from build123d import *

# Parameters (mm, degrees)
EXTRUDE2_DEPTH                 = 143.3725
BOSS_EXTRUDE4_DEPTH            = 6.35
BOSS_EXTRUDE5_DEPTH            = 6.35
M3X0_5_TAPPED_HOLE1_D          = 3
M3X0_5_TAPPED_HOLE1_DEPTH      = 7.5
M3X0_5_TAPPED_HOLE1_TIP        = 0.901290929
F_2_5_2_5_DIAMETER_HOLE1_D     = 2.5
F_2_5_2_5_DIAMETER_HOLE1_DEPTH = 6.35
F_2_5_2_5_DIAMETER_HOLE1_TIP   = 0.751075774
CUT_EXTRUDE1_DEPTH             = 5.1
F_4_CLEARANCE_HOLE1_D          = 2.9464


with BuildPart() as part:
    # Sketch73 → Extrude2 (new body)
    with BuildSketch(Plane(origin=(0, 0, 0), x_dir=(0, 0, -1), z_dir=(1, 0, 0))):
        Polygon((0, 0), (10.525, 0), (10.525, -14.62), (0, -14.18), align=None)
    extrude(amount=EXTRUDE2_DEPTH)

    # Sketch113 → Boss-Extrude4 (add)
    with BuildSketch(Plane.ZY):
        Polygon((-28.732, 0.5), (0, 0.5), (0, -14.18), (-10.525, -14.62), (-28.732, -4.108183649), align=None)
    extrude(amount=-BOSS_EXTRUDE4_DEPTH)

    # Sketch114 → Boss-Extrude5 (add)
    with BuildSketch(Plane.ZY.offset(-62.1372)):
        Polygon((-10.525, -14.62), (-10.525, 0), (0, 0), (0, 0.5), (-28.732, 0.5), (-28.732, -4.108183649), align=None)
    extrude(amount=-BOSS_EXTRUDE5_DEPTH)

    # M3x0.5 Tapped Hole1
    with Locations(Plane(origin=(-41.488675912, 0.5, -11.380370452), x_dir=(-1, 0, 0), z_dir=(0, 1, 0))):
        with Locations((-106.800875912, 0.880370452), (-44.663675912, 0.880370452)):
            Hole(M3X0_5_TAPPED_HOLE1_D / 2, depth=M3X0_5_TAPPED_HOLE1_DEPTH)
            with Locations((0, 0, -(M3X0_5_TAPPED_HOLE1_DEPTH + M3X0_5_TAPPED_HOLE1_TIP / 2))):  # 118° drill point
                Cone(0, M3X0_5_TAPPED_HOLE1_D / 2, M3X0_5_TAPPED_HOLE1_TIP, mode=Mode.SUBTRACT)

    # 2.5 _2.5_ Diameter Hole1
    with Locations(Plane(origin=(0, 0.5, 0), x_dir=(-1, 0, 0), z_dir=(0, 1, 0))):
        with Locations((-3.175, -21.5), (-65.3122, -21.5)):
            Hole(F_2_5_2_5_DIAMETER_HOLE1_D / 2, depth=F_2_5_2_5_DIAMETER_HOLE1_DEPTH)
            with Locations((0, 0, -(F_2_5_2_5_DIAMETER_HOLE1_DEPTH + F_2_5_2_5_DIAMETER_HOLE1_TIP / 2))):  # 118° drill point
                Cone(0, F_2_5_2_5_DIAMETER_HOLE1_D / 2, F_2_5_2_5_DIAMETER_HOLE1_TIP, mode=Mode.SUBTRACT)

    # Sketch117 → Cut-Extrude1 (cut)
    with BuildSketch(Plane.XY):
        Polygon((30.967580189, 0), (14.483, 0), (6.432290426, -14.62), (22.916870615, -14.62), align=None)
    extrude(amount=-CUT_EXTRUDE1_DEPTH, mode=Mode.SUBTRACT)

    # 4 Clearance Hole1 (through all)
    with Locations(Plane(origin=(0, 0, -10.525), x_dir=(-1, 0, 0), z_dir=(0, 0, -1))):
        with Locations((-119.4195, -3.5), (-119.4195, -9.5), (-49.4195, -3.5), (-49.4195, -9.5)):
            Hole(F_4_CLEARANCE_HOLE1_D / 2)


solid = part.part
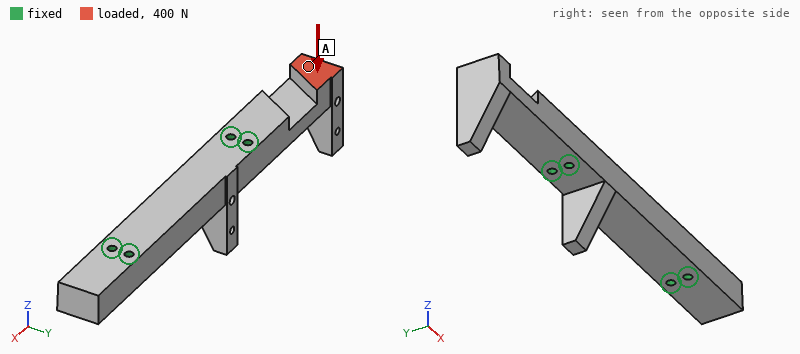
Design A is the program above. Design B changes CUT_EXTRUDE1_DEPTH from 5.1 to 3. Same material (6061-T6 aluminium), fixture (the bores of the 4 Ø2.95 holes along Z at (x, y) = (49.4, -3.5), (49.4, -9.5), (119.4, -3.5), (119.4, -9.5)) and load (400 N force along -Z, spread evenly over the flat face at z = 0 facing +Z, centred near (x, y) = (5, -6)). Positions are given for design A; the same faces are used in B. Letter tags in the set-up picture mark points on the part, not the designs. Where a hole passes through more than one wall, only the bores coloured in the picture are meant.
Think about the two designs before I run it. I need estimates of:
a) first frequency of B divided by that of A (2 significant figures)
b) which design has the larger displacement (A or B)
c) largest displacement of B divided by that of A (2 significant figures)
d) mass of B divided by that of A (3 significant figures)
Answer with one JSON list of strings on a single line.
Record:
["1.2", "A", "0.62", "1.02"]
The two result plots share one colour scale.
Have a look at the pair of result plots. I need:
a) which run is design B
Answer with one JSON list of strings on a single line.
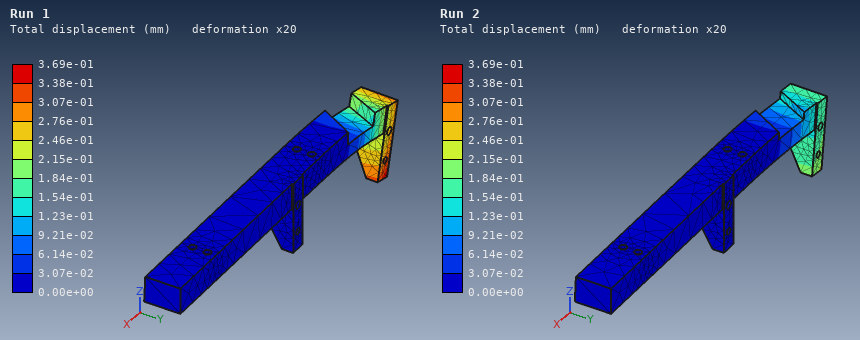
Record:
["Run 2"]
